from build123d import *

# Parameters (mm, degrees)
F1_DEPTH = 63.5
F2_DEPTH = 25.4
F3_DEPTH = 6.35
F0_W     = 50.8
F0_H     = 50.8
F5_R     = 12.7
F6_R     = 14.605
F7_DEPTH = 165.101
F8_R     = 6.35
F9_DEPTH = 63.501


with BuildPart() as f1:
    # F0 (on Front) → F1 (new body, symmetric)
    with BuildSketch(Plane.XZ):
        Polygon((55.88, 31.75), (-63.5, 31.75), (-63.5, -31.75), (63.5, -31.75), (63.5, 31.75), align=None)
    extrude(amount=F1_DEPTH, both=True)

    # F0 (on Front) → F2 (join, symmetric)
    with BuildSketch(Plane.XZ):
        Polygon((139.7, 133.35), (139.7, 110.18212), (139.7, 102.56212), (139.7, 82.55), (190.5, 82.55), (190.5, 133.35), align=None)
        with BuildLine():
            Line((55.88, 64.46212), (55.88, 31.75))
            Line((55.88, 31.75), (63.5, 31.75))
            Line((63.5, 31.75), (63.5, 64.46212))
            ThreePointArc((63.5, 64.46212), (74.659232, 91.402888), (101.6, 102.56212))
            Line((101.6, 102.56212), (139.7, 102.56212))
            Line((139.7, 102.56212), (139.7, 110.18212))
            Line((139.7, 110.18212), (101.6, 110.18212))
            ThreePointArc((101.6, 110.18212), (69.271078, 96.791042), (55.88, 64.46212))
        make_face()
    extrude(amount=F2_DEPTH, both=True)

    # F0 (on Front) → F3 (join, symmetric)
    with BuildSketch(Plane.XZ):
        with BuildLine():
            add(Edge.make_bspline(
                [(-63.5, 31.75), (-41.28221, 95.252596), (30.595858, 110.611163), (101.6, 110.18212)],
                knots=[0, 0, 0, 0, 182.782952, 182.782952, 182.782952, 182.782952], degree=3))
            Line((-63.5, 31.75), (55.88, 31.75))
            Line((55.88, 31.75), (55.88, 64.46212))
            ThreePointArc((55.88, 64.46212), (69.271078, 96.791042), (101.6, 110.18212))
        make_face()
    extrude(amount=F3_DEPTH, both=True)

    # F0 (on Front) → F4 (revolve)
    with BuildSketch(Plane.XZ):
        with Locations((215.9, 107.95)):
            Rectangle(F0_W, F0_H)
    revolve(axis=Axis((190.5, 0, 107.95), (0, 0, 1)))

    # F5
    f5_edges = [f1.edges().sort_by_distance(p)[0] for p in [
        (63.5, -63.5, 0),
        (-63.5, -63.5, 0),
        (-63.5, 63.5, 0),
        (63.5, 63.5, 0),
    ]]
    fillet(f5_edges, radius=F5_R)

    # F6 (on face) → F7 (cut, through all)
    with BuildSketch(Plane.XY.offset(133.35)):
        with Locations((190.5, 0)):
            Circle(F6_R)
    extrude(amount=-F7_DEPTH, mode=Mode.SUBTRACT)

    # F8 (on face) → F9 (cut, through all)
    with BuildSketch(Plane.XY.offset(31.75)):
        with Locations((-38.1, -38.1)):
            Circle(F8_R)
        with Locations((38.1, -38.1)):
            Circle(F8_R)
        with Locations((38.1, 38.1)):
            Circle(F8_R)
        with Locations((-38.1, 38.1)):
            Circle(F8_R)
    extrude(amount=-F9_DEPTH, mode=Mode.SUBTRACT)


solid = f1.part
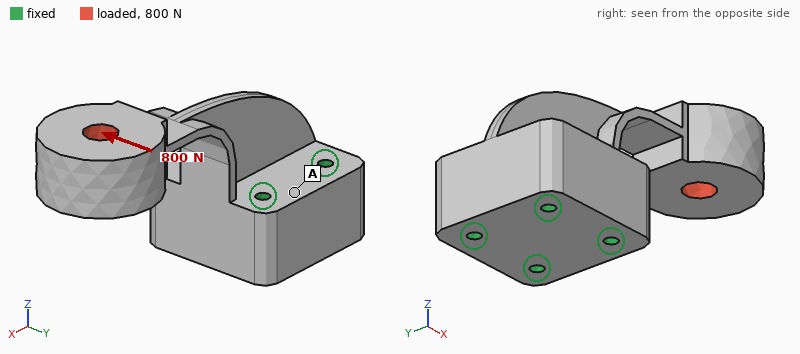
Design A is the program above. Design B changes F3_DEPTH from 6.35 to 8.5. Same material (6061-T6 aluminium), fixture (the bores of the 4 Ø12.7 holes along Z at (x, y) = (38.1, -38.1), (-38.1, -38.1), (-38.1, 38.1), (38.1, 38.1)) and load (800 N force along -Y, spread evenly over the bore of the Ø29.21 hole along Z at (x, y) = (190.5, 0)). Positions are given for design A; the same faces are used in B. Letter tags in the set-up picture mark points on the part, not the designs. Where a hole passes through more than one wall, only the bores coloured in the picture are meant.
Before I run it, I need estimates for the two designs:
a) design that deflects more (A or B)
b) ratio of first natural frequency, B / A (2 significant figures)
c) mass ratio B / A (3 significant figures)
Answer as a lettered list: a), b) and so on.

a) A
b) 1.0
c) 1.02
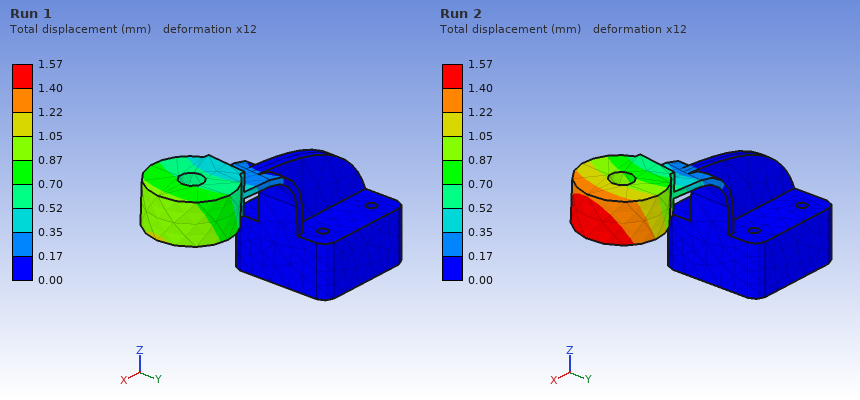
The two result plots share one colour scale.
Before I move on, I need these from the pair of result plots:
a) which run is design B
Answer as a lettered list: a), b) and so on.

a) Run 1
